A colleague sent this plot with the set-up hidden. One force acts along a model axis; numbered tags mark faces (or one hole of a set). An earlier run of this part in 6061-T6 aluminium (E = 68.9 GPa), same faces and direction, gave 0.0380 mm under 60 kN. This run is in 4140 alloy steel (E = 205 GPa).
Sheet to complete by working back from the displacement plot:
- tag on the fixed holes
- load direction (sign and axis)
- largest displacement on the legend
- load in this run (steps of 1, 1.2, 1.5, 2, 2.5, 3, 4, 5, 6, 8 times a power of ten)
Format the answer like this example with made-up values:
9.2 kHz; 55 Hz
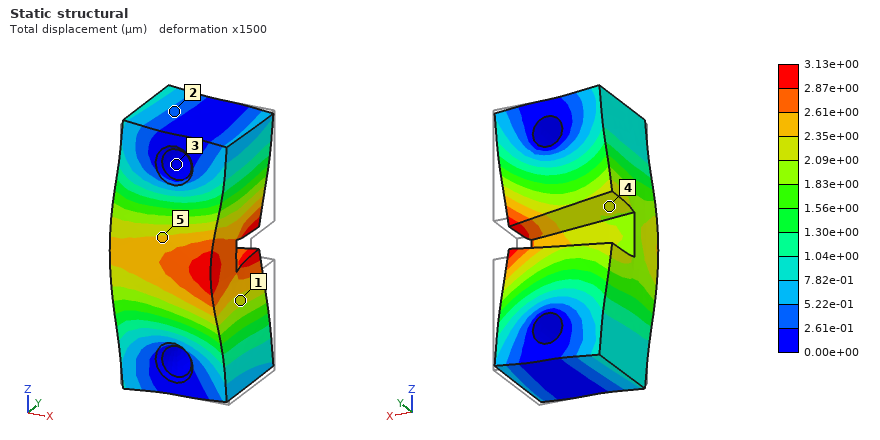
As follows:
3; -X; 3.13e+00 µm; 15 kN
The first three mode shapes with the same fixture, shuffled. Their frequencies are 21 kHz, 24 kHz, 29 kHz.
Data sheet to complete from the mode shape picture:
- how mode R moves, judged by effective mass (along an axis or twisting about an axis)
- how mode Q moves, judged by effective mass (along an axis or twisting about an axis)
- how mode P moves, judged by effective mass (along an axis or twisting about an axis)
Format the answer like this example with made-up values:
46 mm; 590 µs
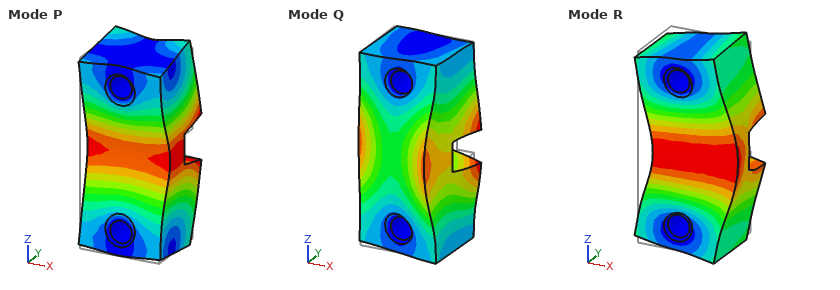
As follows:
along X; twisting about Z; along Y
